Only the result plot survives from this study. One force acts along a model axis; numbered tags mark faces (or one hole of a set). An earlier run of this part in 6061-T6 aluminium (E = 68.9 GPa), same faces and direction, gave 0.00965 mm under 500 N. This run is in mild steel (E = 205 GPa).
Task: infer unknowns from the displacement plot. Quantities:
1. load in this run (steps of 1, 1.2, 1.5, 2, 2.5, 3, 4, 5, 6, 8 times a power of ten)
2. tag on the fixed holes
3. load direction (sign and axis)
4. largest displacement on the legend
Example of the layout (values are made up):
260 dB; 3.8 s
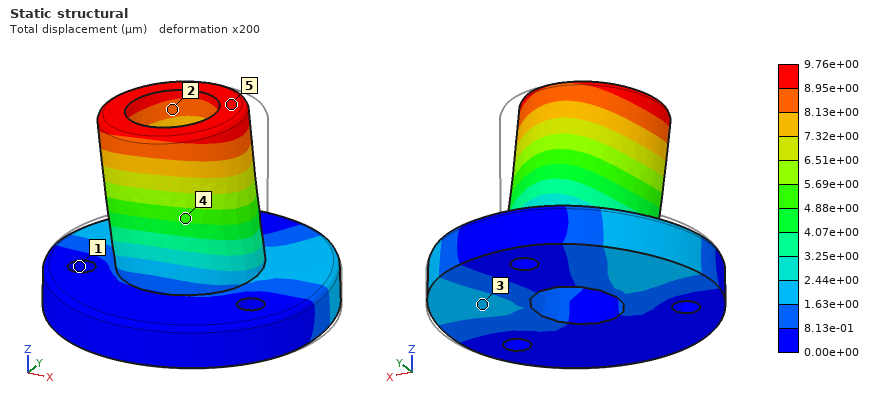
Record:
1.5 kN; 1; -X; 9.76e+00 µm
